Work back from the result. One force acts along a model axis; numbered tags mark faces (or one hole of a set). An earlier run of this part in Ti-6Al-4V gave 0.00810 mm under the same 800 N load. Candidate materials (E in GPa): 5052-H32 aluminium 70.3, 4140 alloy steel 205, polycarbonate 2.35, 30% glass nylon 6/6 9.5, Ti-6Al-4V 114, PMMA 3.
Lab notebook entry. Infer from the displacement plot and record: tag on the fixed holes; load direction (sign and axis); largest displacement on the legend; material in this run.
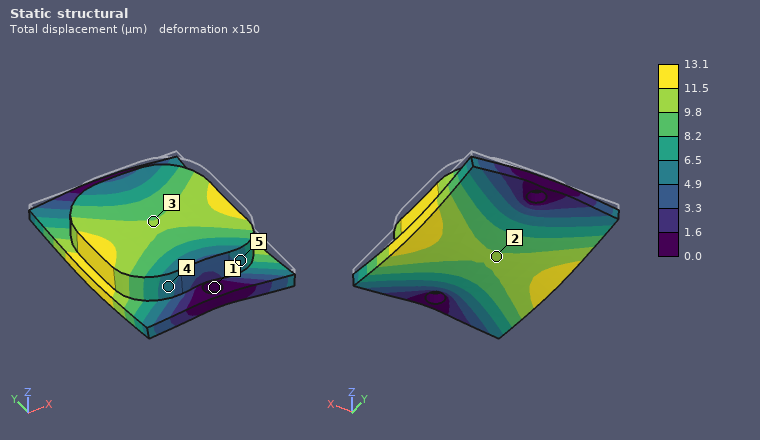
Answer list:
1
-Z
13.1 µm
5052-H32 aluminium
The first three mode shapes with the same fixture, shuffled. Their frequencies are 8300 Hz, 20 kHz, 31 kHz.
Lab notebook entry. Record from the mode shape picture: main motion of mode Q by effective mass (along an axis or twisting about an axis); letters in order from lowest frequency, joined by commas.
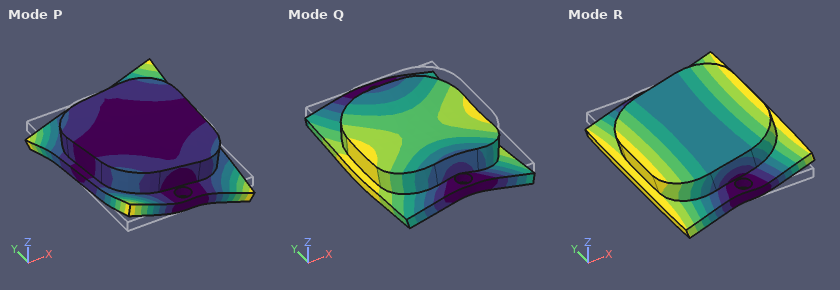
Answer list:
along Z
R, Q, P
